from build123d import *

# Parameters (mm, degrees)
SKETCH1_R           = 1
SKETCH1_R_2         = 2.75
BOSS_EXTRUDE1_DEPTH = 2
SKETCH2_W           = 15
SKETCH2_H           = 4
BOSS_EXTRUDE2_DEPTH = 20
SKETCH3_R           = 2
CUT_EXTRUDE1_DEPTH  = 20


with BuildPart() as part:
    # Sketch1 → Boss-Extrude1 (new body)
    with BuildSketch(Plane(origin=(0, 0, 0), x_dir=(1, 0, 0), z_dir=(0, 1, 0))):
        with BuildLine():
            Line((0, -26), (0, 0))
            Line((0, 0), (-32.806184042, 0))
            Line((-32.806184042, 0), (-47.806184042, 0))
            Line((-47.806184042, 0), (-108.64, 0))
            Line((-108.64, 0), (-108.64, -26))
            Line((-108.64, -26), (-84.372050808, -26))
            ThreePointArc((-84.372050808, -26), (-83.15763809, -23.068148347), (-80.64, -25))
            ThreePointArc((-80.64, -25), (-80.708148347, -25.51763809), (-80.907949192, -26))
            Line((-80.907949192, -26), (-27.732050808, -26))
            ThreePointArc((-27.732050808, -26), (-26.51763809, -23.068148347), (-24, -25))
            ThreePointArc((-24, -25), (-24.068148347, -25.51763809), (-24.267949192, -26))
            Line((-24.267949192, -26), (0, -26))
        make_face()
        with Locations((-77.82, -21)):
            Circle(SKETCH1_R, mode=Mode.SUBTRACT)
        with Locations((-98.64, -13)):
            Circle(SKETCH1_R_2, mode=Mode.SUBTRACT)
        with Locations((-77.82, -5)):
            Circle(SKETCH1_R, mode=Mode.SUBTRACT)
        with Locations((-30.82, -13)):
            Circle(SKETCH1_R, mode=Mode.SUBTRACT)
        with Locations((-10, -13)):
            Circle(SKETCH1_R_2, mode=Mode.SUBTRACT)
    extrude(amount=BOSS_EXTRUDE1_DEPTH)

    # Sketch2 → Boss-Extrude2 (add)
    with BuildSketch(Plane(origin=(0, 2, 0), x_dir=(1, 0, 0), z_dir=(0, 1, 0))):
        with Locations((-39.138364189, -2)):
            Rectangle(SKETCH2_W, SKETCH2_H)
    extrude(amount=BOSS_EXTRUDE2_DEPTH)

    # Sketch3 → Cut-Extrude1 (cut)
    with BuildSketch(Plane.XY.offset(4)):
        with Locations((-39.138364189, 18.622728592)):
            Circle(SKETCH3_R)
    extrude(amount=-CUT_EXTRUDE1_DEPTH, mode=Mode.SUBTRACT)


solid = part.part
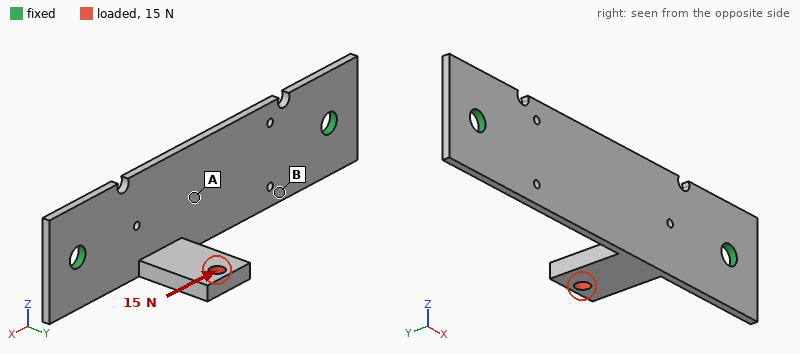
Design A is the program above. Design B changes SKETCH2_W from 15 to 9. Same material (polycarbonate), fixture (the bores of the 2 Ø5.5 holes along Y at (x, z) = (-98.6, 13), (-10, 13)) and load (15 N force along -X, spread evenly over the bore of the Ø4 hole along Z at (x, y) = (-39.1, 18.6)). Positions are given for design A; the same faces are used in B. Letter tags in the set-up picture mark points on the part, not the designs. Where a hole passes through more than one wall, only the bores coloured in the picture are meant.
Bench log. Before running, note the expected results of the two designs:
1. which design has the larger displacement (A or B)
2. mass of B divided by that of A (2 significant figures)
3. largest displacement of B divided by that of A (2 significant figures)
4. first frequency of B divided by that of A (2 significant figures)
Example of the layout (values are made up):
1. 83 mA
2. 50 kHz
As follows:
1. B
2. 0.93
3. 1.3
4. 1.1
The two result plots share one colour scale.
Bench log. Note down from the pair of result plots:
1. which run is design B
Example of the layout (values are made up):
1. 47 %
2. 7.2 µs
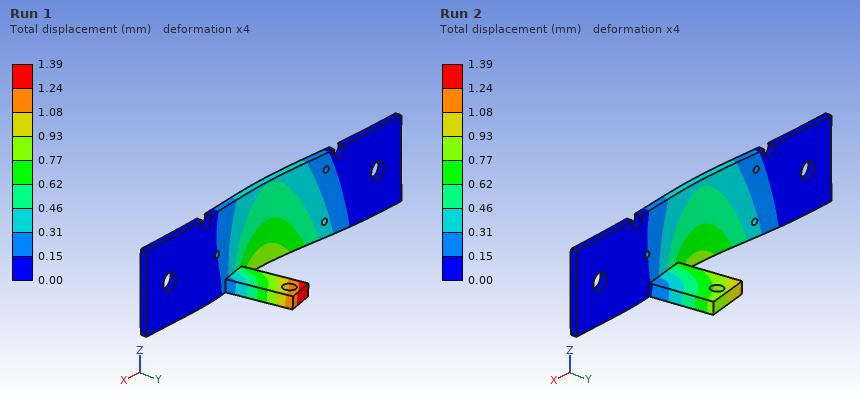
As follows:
1. Run 1
